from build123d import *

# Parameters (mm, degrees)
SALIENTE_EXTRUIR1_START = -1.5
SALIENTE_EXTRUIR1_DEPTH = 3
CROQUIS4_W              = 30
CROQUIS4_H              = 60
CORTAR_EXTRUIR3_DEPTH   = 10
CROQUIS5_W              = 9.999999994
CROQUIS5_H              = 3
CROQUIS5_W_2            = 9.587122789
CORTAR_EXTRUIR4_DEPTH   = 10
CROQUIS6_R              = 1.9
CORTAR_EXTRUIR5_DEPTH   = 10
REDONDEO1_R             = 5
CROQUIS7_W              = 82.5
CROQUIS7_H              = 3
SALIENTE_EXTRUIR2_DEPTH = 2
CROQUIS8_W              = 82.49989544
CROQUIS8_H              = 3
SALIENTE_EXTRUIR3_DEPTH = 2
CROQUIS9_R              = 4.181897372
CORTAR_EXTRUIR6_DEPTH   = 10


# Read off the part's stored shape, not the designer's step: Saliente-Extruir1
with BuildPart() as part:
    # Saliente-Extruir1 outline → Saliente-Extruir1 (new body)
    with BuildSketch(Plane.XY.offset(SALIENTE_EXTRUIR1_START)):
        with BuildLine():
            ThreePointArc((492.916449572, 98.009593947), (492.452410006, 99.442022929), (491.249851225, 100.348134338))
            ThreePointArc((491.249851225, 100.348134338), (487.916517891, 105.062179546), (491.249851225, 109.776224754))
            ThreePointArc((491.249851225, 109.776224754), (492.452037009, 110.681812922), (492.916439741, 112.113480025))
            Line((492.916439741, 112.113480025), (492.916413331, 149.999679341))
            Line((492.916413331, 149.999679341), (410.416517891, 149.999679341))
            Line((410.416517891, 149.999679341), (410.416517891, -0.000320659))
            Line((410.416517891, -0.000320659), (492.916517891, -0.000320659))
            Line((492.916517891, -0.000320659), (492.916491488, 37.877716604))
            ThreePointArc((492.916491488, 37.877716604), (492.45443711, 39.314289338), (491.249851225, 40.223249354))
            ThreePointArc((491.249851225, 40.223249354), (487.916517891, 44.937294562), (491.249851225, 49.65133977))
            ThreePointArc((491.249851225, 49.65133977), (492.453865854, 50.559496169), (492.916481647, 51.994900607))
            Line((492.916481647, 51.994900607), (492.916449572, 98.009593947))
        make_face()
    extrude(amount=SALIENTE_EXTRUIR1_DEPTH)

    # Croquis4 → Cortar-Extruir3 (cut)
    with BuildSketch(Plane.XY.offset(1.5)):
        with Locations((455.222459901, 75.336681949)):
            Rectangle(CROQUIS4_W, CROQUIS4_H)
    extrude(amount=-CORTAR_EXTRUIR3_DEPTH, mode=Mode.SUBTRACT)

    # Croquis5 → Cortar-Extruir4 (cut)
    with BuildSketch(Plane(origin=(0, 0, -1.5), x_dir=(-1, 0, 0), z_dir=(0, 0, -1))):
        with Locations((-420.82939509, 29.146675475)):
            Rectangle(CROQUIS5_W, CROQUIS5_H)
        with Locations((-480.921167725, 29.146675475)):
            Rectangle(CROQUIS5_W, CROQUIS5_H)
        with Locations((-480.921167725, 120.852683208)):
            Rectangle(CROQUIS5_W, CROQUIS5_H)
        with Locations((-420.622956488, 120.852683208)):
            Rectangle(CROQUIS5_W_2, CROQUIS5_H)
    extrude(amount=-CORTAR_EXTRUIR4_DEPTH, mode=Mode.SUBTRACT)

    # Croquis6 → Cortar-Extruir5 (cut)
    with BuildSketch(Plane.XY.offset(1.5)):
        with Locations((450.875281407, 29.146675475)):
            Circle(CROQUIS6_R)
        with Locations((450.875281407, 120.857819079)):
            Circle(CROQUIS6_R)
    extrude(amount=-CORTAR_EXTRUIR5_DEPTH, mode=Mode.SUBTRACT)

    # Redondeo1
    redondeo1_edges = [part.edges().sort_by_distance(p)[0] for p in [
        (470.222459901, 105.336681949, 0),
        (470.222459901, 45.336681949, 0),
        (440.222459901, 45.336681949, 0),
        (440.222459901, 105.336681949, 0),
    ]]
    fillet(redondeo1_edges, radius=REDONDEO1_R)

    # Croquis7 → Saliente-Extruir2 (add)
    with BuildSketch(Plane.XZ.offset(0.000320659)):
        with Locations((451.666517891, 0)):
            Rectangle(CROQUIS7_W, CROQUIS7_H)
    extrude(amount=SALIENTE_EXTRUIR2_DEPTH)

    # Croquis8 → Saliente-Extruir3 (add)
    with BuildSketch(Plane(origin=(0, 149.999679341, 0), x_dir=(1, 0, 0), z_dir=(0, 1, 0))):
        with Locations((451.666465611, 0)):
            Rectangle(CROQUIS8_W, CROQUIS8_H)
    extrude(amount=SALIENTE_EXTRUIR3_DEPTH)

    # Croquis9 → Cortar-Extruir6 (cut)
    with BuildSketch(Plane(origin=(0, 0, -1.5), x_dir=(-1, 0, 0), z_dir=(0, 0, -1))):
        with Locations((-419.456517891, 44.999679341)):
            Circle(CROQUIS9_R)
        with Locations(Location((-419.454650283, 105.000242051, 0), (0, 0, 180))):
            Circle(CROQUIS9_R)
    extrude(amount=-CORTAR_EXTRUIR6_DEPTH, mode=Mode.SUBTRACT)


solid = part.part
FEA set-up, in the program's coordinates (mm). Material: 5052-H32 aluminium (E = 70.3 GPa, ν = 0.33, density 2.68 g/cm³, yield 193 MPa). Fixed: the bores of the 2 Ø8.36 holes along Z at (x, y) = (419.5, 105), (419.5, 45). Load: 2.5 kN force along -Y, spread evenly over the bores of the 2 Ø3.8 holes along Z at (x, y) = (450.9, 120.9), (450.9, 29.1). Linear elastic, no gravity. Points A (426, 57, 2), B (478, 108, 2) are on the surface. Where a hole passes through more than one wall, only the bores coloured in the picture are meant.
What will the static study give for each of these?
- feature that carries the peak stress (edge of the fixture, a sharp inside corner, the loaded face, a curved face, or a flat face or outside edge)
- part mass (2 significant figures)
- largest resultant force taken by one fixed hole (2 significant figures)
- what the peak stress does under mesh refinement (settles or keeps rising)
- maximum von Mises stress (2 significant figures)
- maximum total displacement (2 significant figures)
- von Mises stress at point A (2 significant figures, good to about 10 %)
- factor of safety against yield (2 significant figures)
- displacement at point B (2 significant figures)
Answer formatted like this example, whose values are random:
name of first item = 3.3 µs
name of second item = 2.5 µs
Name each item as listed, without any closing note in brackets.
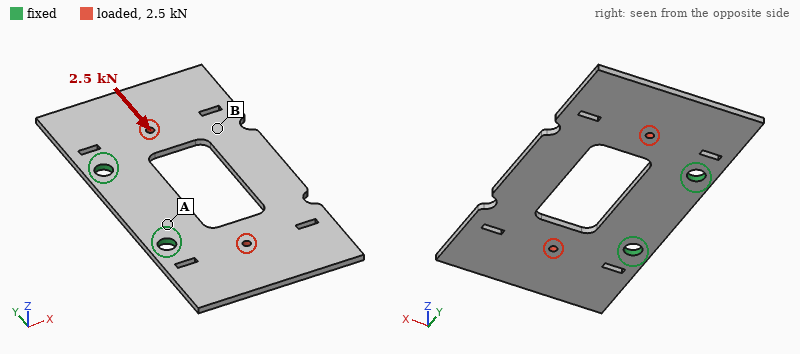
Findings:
feature that carries the peak stress = a curved face
part mass = 85 g
largest resultant force taken by one fixed hole = 1.6 kN
what the peak stress does under mesh refinement = settles
maximum von Mises stress = 120 MPa
maximum total displacement = 0.11 mm
von Mises stress at point A = 26 MPa
factor of safety against yield = 1.6
displacement at point B = 0.079 mm
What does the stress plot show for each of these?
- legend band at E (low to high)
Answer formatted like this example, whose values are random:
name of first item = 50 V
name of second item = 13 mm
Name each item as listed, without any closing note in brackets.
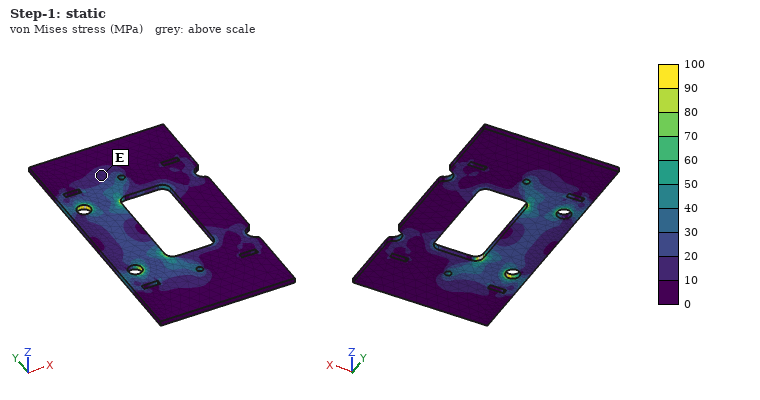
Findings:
legend band at E = 10 to 20 MPa
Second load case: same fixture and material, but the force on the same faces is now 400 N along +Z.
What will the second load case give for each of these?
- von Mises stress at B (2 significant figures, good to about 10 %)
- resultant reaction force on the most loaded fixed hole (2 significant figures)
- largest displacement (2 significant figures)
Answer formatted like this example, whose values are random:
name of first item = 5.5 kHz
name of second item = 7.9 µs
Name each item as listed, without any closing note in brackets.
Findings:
von Mises stress at B = 13 MPa
resultant reaction force on the most loaded fixed hole = 200 N
largest displacement = 1.2 mm
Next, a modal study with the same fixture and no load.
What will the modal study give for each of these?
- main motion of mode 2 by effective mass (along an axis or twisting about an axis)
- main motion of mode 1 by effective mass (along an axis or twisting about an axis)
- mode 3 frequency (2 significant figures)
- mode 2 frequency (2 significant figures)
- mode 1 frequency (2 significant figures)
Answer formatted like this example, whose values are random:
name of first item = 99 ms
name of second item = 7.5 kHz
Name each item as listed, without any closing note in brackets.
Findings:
main motion of mode 2 by effective mass = twisting about X
main motion of mode 1 by effective mass = along Z
mode 3 frequency = 800 Hz
mode 2 frequency = 450 Hz
mode 1 frequency = 350 Hz
